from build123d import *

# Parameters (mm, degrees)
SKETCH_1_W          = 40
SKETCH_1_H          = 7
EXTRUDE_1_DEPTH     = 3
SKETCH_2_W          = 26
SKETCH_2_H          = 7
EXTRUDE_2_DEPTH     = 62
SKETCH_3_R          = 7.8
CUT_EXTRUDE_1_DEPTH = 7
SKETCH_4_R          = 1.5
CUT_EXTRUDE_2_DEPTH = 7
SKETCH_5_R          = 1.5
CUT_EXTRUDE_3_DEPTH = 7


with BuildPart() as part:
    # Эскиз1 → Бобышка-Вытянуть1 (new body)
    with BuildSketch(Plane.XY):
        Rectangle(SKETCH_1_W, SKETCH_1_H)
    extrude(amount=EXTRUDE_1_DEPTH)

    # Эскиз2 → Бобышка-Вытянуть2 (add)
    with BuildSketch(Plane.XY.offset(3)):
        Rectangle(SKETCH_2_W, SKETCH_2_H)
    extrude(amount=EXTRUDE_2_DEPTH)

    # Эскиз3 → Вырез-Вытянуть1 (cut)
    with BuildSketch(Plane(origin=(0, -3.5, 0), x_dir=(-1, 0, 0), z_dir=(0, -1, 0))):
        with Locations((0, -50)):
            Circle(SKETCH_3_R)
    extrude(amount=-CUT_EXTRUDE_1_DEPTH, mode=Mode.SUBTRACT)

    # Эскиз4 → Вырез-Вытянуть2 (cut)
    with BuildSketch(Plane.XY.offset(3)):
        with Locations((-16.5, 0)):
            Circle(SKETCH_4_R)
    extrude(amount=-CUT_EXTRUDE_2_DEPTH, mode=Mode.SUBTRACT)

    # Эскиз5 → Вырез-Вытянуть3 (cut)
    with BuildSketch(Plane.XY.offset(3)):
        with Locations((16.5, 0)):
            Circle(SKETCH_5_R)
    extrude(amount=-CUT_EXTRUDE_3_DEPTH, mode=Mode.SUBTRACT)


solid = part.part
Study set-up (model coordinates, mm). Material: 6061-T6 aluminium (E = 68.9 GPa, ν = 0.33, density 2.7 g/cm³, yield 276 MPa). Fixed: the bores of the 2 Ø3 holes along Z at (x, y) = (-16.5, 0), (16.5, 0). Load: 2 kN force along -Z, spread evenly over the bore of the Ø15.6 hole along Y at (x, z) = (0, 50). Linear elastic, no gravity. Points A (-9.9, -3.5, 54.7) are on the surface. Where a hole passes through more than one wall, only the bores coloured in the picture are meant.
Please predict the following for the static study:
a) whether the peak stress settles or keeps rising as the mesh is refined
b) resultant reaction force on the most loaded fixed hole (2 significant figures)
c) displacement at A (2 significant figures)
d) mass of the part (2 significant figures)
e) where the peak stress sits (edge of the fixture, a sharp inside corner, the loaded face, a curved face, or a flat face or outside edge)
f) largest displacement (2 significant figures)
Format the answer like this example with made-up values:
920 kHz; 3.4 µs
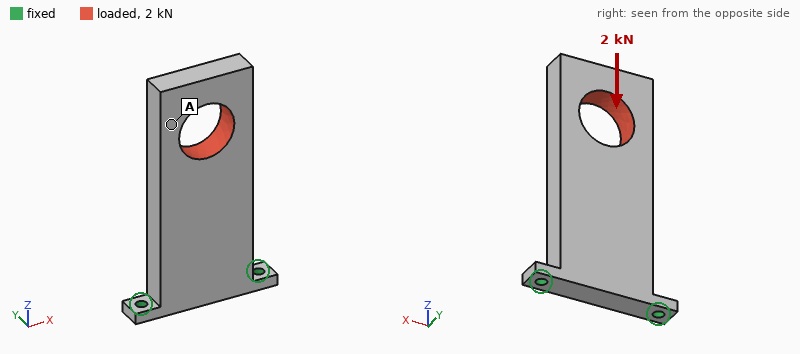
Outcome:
keeps rising; 1.1 kN; 26 µm; 29 g; edge of the fixture; 30 µm
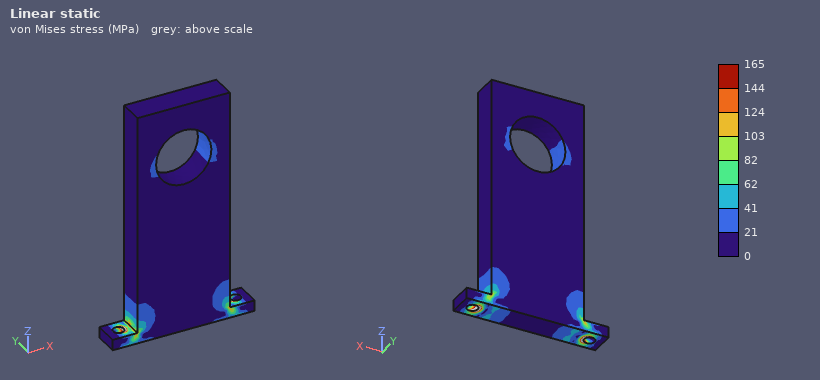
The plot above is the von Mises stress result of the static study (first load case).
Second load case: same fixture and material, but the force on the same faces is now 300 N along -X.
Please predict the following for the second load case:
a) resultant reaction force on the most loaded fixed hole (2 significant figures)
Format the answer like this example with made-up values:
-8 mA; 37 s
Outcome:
550 N
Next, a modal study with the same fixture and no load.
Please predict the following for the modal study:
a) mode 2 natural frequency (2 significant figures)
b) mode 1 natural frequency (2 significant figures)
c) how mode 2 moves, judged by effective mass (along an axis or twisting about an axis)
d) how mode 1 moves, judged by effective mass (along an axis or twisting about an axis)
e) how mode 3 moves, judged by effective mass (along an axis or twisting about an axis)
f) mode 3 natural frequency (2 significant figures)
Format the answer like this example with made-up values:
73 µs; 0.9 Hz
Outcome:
3400 Hz; 700 Hz; along X; along Y; twisting about Z; 5600 Hz
